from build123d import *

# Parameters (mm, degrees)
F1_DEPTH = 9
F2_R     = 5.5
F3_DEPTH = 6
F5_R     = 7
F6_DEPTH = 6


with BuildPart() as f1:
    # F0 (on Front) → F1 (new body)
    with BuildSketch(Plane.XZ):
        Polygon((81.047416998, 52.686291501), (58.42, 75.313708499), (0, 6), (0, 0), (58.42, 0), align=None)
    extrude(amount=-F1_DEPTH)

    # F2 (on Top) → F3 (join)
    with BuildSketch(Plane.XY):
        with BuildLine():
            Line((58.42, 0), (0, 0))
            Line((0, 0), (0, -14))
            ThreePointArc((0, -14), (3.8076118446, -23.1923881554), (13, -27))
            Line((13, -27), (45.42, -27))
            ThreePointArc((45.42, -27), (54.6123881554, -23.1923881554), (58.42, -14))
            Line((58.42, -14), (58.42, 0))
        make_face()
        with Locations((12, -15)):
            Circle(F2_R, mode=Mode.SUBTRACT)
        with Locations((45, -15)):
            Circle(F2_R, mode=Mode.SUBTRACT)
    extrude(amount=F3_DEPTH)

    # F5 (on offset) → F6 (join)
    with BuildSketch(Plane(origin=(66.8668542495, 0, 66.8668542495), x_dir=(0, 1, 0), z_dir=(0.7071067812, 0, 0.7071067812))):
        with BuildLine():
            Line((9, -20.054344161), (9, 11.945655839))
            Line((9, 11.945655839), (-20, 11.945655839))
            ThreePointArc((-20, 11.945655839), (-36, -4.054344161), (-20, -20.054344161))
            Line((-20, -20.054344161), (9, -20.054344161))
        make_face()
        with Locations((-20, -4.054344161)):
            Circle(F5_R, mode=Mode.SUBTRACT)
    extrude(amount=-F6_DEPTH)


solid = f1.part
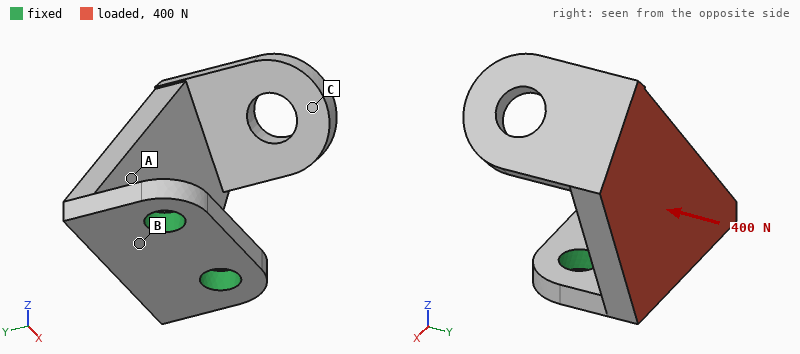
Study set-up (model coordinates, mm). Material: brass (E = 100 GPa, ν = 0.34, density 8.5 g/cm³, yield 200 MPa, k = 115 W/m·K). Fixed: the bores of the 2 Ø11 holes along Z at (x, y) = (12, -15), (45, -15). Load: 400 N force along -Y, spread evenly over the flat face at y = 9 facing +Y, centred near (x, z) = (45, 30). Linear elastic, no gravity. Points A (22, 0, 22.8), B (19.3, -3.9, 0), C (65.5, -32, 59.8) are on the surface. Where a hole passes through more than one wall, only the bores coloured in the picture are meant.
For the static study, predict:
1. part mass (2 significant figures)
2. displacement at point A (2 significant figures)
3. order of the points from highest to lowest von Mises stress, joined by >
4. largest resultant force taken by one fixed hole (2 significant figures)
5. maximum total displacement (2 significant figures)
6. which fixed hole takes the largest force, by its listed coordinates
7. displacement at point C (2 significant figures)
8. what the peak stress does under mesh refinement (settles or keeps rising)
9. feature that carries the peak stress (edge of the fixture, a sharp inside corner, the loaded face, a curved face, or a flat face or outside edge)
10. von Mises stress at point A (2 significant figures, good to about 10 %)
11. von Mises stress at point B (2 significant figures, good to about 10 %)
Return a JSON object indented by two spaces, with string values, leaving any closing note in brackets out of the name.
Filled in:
{
  "part mass": "360 g",
  "displacement at point A": "0.029 mm",
  "order of the points from highest to lowest von Mises stress, joined by >": "B > A > C",
  "largest resultant force taken by one fixed hole": "370 N",
  "maximum total displacement": "0.16 mm",
  "which fixed hole takes the largest force, by its listed coordinates": "(45, -15)",
  "displacement at point C": "0.14 mm",
  "what the peak stress does under mesh refinement": "keeps rising",
  "feature that carries the peak stress": "edge of the fixture",
  "von Mises stress at point A": "10 MPa",
  "von Mises stress at point B": "23 MPa"
}
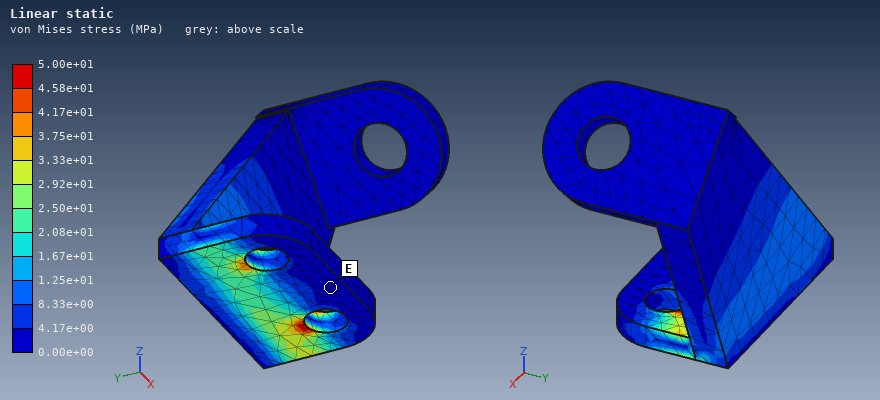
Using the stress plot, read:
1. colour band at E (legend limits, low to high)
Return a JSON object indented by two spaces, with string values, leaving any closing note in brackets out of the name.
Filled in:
{
  "colour band at E": "0.00e+00 to 4.17e+00 MPa"
}
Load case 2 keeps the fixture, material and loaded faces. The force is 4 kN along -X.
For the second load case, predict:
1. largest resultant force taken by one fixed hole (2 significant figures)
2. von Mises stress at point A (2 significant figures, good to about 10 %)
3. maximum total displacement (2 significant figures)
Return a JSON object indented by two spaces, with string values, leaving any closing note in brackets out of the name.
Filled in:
{
  "largest resultant force taken by one fixed hole": "4.1 kN",
  "von Mises stress at point A": "33 MPa",
  "maximum total displacement": "0.17 mm"
}
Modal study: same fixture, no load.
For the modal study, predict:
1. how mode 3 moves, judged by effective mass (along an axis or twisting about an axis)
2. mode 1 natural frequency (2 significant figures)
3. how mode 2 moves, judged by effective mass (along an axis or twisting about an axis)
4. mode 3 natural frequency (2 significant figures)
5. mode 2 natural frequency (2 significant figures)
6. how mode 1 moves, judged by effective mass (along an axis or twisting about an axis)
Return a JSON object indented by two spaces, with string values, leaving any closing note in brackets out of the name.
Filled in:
{
  "how mode 3 moves, judged by effective mass": "along Z",
  "mode 1 natural frequency": "520 Hz",
  "how mode 2 moves, judged by effective mass": "along X",
  "mode 3 natural frequency": "1800 Hz",
  "mode 2 natural frequency": "1200 Hz",
  "how mode 1 moves, judged by effective mass": "along Y"
}
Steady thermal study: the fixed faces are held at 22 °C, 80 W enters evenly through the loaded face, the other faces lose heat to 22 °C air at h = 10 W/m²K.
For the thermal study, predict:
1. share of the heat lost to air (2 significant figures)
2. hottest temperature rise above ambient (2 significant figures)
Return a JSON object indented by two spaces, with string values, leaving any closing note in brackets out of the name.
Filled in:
{
  "share of the heat lost to air": "5.8 %",
  "hottest temperature rise above ambient": "74 K"
}
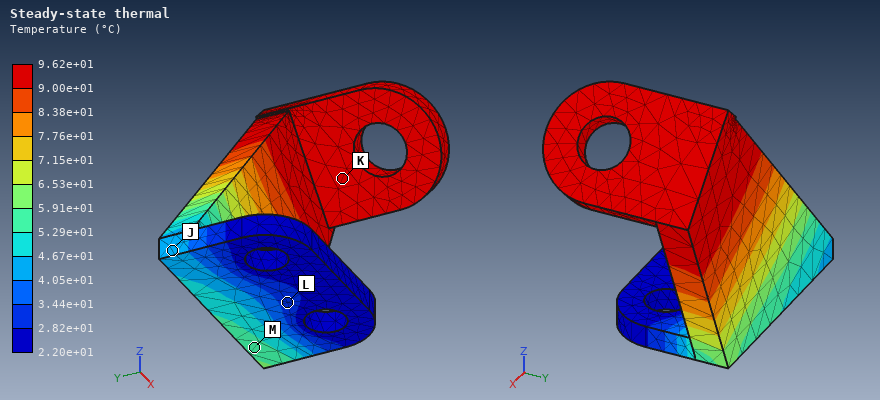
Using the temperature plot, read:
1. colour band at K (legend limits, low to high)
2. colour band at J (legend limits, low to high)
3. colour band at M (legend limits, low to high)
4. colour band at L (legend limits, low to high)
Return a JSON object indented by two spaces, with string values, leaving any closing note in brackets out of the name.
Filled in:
{
  "colour band at K": "9.00e+01 to 9.62e+01 °C",
  "colour band at J": "4.05e+01 to 4.67e+01 °C",
  "colour band at M": "5.29e+01 to 5.91e+01 °C",
  "colour band at L": "2.82e+01 to 3.44e+01 °C"
}
